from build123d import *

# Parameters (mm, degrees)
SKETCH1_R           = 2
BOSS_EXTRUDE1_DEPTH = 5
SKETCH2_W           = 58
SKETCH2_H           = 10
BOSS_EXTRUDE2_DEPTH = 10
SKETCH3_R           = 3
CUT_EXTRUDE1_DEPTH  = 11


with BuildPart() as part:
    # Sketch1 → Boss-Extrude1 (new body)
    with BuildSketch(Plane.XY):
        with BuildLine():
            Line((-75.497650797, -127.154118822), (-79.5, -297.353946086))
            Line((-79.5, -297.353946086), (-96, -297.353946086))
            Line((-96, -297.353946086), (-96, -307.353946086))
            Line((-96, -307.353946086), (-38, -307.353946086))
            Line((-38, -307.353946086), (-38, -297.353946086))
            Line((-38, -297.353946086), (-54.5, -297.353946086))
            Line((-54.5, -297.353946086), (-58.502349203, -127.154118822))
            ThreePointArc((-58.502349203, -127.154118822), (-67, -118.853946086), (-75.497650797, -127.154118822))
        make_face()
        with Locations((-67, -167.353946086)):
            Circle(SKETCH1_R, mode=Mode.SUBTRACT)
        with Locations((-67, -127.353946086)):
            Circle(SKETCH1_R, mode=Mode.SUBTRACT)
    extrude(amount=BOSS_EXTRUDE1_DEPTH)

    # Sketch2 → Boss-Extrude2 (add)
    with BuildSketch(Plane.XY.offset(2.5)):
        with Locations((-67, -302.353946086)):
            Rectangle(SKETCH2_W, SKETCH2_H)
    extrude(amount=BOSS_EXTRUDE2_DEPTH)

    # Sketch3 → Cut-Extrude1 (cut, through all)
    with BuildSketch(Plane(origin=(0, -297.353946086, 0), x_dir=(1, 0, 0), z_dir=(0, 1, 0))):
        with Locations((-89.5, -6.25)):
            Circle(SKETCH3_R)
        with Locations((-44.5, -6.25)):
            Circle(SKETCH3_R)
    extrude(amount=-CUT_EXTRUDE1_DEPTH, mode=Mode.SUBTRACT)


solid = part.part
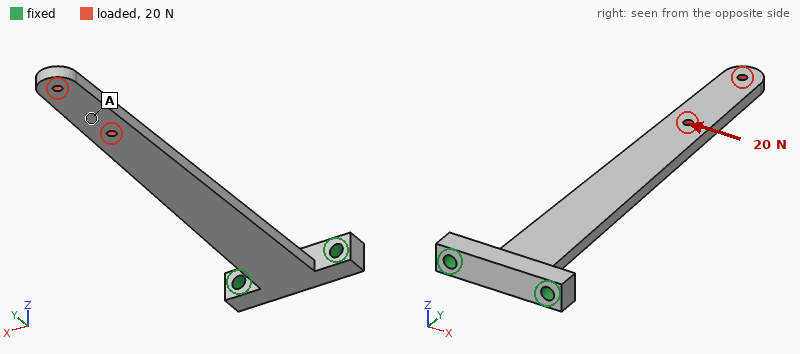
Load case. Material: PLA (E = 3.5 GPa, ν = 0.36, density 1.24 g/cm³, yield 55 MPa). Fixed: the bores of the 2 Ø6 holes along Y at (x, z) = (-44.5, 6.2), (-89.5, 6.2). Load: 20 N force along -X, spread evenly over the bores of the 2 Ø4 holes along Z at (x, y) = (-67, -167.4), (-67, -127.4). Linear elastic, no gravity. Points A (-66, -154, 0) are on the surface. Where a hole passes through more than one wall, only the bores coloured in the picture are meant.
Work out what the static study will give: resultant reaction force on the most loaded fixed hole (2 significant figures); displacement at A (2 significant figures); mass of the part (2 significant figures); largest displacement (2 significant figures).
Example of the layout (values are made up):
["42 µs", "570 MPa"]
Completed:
["95 N", "1.4 mm", "31 g", "1.9 mm"]
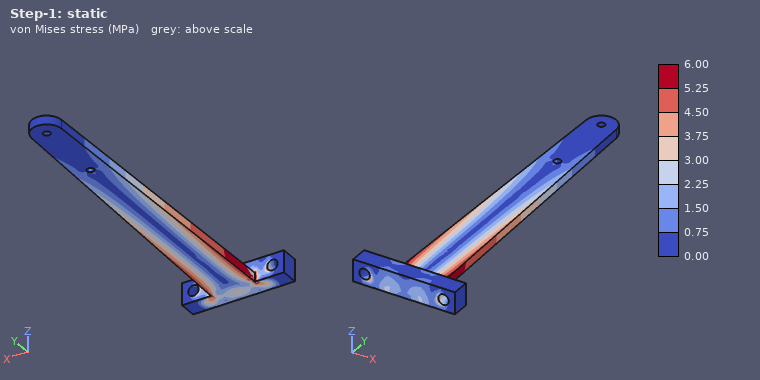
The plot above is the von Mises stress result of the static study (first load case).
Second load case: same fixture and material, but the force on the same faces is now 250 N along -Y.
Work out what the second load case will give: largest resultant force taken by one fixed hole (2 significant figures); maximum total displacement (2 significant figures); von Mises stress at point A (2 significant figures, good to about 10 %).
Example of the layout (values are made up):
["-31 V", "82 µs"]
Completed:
["130 N", "0.42 mm", "1.2 MPa"]
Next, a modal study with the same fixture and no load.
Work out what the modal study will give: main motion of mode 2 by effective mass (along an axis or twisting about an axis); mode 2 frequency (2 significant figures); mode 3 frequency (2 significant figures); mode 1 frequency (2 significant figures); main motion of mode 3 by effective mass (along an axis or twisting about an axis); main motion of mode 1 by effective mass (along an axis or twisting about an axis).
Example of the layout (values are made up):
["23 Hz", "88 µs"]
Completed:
["along X", "210 Hz", "270 Hz", "48 Hz", "along Z", "along Z"]
